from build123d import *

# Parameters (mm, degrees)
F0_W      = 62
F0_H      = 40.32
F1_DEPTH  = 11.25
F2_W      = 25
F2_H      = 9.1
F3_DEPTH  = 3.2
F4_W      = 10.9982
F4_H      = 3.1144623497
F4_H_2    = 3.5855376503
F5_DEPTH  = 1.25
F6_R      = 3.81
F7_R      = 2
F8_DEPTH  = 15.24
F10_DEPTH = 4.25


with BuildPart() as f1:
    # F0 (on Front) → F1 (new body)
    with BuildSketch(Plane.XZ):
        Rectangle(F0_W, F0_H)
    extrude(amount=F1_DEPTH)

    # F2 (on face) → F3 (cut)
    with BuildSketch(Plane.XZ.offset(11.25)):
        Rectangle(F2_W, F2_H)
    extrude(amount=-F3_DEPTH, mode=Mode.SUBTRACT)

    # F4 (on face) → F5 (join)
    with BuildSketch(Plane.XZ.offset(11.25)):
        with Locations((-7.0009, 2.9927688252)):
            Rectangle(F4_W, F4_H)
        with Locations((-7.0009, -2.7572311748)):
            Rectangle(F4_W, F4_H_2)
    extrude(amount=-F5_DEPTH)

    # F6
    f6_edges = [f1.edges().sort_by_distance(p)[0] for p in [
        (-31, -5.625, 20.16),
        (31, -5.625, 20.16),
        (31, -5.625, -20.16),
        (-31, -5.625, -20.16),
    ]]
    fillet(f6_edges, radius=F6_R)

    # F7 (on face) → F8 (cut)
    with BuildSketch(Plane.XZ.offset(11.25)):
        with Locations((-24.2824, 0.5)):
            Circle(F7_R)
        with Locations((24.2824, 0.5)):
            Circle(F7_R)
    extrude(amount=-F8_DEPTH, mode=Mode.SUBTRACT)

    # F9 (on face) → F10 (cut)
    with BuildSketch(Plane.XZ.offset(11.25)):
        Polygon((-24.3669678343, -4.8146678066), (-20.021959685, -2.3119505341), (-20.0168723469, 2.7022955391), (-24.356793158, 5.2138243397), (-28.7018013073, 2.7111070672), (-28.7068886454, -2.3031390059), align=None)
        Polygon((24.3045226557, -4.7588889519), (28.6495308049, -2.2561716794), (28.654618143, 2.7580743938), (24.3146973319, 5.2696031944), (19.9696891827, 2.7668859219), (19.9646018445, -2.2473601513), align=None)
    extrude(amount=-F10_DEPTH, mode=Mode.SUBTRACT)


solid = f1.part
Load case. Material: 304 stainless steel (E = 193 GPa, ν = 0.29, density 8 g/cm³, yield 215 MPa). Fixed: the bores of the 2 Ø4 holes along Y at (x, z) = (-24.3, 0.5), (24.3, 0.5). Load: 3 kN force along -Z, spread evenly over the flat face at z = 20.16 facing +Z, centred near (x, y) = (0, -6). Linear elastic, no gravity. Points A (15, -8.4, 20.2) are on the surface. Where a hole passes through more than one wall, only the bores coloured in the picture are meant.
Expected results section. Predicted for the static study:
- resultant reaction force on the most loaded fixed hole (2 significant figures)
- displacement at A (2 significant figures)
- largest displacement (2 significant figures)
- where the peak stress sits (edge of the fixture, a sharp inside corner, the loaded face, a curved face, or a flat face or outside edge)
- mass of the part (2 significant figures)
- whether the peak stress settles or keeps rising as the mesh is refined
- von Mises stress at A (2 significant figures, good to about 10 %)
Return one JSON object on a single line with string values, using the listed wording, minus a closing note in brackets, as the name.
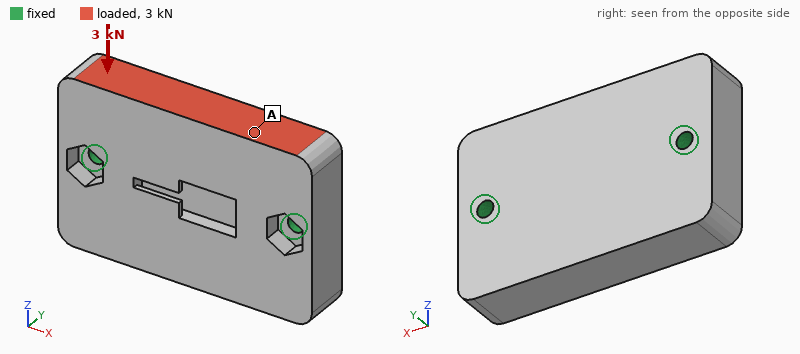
{"resultant reaction force on the most loaded fixed hole": "1.5 kN", "displacement at A": "3.0 µm", "largest displacement": "3.6 µm", "where the peak stress sits": "edge of the fixture", "mass of the part": "210 g", "whether the peak stress settles or keeps rising as the mesh is refined": "keeps rising", "von Mises stress at A": "4.4 MPa"}
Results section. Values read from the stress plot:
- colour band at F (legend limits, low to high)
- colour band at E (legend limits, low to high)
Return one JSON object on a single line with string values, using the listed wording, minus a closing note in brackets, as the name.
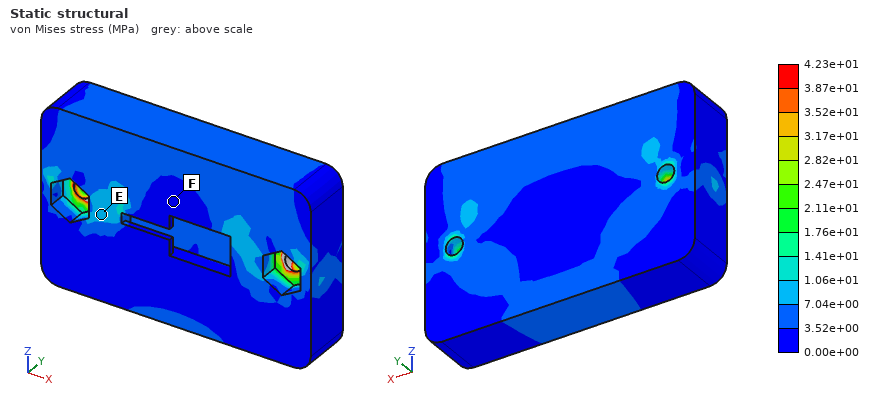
{"colour band at F": "0.00e+00 to 3.52e+00 MPa", "colour band at E": "7.04e+00 to 1.06e+01 MPa"}
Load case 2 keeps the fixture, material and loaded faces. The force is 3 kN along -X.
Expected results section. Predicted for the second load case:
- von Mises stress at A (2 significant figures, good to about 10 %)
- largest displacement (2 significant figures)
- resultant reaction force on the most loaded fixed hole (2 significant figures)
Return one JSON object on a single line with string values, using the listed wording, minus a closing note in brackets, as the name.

{"von Mises stress at A": "9.5 MPa", "largest displacement": "2.6 µm", "resultant reaction force on the most loaded fixed hole": "1.9 kN"}
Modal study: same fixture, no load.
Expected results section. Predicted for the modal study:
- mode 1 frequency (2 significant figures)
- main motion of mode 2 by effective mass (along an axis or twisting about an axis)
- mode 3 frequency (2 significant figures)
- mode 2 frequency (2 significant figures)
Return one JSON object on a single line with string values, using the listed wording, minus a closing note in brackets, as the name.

{"mode 1 frequency": "6600 Hz", "main motion of mode 2 by effective mass": "along Y", "mode 3 frequency": "14 kHz", "mode 2 frequency": "10 kHz"}
